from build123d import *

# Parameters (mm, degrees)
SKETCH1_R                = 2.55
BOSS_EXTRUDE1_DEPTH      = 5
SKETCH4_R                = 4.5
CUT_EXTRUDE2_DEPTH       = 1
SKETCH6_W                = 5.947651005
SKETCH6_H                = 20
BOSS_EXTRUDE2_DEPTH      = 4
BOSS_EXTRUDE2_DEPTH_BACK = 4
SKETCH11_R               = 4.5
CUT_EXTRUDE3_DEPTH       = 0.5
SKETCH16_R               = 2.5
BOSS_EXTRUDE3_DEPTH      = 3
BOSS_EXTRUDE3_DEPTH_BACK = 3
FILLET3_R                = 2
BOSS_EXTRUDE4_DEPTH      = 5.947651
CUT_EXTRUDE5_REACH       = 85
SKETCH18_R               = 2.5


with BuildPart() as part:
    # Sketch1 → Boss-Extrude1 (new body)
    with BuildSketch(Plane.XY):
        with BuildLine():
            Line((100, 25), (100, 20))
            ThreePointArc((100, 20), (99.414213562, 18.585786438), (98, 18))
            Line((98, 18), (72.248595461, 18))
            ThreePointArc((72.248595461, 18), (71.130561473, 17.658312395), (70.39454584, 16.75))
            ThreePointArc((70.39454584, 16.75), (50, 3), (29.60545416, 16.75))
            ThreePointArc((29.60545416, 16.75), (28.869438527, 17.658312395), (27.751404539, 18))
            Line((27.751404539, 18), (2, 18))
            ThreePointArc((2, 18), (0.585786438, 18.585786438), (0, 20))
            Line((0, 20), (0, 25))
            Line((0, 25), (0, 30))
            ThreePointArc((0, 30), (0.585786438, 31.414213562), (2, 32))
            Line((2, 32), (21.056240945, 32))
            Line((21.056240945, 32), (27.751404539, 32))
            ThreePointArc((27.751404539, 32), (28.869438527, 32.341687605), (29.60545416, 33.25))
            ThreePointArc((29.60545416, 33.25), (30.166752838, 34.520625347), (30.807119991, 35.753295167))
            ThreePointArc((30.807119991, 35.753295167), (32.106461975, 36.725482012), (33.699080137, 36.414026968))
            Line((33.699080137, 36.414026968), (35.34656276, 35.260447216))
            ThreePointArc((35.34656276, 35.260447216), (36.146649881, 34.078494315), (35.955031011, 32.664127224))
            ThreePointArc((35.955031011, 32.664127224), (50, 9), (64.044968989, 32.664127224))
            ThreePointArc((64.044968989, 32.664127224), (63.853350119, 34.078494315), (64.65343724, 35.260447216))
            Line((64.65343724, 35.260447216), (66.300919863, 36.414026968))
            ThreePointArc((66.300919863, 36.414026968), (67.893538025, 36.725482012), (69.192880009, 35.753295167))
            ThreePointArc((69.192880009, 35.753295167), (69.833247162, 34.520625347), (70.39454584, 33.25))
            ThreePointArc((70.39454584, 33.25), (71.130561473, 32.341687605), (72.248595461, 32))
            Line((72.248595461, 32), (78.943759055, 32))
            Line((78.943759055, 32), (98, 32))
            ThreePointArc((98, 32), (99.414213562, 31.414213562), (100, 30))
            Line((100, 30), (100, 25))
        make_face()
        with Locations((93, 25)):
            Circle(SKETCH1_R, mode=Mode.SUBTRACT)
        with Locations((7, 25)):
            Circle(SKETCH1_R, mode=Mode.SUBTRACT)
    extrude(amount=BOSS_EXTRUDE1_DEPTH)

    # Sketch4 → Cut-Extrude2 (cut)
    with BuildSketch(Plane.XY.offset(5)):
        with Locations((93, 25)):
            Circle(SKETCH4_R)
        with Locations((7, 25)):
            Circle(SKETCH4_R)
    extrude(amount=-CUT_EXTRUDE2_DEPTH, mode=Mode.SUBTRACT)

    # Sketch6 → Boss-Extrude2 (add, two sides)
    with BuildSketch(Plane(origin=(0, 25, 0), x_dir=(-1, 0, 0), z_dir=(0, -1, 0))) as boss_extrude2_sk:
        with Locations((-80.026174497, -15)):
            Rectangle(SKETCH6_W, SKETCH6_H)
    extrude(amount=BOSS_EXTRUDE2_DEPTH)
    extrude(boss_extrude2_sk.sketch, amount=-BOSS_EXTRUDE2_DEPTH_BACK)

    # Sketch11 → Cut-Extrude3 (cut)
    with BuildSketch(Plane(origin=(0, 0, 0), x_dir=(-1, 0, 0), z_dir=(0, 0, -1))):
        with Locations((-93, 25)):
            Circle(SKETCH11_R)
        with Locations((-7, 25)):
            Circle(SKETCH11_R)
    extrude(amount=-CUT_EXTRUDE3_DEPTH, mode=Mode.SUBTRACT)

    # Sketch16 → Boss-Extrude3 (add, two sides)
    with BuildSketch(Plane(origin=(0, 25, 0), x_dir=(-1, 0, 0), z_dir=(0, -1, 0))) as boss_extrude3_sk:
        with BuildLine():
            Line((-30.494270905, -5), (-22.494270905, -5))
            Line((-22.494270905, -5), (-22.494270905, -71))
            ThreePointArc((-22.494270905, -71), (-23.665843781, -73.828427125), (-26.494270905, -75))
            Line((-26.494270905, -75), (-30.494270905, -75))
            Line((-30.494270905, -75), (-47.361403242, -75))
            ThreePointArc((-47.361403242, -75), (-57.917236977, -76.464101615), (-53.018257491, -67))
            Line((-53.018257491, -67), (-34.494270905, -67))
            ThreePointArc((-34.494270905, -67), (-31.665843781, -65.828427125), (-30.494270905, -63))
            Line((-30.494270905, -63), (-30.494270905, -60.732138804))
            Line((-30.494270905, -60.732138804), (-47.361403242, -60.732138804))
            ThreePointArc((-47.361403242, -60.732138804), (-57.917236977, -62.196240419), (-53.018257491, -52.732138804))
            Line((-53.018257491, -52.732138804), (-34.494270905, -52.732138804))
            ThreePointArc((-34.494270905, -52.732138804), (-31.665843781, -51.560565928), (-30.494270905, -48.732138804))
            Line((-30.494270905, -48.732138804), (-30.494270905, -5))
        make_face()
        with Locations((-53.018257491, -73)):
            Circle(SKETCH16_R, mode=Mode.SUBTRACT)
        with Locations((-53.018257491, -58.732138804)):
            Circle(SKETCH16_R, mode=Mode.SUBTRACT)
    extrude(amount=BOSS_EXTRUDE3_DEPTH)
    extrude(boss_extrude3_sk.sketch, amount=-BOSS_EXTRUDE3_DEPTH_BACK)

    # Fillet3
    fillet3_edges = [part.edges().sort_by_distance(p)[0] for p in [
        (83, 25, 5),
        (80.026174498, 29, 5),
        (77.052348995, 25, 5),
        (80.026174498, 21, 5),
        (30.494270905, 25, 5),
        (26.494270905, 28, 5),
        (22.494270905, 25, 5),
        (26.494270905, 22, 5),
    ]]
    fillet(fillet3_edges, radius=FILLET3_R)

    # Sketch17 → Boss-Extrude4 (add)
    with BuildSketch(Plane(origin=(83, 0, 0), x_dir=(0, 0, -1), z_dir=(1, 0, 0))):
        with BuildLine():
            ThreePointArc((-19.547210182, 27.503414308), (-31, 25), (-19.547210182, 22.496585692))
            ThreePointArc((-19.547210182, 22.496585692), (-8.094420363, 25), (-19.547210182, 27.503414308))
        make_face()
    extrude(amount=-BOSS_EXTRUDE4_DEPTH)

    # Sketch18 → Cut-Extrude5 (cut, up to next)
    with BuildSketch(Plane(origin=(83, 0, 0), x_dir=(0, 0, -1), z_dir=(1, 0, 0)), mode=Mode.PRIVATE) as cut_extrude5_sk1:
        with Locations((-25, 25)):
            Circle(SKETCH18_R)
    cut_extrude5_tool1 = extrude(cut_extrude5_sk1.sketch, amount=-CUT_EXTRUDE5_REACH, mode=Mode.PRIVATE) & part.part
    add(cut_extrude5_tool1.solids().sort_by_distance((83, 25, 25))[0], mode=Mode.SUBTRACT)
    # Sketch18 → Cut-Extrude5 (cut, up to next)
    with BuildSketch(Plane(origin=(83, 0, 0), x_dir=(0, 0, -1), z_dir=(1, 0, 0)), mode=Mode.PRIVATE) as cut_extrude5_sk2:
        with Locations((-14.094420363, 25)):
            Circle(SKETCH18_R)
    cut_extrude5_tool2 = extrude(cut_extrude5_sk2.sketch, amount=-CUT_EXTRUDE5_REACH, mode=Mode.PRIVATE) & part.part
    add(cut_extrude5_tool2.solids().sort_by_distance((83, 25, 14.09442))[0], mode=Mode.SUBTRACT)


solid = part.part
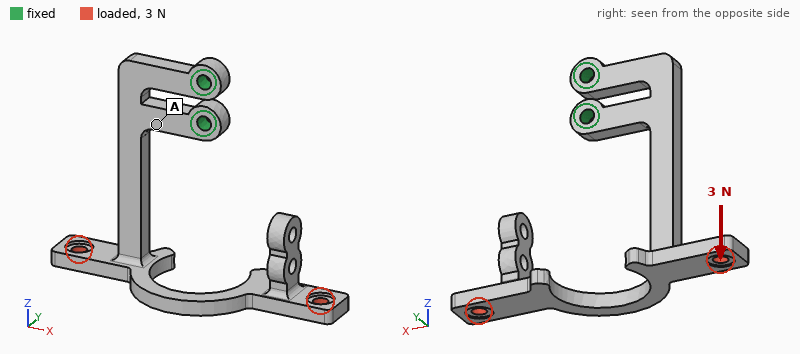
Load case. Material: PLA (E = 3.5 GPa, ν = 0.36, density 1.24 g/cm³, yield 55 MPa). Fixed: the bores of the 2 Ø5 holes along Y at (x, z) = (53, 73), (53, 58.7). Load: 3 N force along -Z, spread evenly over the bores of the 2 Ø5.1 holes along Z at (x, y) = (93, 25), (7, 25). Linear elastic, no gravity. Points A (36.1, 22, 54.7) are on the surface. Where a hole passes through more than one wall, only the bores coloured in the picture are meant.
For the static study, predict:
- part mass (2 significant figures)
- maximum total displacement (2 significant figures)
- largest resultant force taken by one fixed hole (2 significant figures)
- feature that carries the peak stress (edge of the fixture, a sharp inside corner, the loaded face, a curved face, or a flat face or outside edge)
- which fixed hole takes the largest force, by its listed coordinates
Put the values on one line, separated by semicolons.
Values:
17 g; 1.4 mm; 3.1 N; a flat face or outside edge; (53, 58.7)
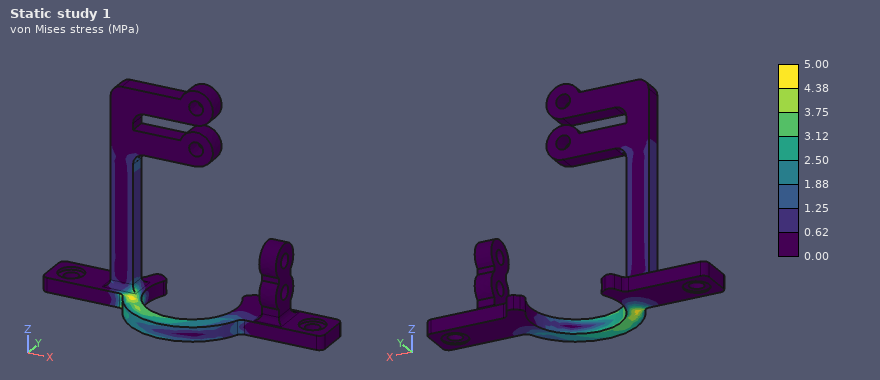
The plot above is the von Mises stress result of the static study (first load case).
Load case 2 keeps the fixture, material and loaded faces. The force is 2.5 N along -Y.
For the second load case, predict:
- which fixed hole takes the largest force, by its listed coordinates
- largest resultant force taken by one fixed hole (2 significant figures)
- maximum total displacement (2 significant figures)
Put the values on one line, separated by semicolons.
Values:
(53, 58.7); 5.7 N; 1.5 mm
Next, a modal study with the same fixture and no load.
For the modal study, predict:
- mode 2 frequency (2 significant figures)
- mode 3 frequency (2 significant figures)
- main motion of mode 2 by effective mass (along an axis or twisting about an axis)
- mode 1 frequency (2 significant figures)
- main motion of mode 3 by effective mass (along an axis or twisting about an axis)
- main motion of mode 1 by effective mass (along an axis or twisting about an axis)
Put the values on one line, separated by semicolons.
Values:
94 Hz; 170 Hz; along Z; 81 Hz; along Y; along Y
